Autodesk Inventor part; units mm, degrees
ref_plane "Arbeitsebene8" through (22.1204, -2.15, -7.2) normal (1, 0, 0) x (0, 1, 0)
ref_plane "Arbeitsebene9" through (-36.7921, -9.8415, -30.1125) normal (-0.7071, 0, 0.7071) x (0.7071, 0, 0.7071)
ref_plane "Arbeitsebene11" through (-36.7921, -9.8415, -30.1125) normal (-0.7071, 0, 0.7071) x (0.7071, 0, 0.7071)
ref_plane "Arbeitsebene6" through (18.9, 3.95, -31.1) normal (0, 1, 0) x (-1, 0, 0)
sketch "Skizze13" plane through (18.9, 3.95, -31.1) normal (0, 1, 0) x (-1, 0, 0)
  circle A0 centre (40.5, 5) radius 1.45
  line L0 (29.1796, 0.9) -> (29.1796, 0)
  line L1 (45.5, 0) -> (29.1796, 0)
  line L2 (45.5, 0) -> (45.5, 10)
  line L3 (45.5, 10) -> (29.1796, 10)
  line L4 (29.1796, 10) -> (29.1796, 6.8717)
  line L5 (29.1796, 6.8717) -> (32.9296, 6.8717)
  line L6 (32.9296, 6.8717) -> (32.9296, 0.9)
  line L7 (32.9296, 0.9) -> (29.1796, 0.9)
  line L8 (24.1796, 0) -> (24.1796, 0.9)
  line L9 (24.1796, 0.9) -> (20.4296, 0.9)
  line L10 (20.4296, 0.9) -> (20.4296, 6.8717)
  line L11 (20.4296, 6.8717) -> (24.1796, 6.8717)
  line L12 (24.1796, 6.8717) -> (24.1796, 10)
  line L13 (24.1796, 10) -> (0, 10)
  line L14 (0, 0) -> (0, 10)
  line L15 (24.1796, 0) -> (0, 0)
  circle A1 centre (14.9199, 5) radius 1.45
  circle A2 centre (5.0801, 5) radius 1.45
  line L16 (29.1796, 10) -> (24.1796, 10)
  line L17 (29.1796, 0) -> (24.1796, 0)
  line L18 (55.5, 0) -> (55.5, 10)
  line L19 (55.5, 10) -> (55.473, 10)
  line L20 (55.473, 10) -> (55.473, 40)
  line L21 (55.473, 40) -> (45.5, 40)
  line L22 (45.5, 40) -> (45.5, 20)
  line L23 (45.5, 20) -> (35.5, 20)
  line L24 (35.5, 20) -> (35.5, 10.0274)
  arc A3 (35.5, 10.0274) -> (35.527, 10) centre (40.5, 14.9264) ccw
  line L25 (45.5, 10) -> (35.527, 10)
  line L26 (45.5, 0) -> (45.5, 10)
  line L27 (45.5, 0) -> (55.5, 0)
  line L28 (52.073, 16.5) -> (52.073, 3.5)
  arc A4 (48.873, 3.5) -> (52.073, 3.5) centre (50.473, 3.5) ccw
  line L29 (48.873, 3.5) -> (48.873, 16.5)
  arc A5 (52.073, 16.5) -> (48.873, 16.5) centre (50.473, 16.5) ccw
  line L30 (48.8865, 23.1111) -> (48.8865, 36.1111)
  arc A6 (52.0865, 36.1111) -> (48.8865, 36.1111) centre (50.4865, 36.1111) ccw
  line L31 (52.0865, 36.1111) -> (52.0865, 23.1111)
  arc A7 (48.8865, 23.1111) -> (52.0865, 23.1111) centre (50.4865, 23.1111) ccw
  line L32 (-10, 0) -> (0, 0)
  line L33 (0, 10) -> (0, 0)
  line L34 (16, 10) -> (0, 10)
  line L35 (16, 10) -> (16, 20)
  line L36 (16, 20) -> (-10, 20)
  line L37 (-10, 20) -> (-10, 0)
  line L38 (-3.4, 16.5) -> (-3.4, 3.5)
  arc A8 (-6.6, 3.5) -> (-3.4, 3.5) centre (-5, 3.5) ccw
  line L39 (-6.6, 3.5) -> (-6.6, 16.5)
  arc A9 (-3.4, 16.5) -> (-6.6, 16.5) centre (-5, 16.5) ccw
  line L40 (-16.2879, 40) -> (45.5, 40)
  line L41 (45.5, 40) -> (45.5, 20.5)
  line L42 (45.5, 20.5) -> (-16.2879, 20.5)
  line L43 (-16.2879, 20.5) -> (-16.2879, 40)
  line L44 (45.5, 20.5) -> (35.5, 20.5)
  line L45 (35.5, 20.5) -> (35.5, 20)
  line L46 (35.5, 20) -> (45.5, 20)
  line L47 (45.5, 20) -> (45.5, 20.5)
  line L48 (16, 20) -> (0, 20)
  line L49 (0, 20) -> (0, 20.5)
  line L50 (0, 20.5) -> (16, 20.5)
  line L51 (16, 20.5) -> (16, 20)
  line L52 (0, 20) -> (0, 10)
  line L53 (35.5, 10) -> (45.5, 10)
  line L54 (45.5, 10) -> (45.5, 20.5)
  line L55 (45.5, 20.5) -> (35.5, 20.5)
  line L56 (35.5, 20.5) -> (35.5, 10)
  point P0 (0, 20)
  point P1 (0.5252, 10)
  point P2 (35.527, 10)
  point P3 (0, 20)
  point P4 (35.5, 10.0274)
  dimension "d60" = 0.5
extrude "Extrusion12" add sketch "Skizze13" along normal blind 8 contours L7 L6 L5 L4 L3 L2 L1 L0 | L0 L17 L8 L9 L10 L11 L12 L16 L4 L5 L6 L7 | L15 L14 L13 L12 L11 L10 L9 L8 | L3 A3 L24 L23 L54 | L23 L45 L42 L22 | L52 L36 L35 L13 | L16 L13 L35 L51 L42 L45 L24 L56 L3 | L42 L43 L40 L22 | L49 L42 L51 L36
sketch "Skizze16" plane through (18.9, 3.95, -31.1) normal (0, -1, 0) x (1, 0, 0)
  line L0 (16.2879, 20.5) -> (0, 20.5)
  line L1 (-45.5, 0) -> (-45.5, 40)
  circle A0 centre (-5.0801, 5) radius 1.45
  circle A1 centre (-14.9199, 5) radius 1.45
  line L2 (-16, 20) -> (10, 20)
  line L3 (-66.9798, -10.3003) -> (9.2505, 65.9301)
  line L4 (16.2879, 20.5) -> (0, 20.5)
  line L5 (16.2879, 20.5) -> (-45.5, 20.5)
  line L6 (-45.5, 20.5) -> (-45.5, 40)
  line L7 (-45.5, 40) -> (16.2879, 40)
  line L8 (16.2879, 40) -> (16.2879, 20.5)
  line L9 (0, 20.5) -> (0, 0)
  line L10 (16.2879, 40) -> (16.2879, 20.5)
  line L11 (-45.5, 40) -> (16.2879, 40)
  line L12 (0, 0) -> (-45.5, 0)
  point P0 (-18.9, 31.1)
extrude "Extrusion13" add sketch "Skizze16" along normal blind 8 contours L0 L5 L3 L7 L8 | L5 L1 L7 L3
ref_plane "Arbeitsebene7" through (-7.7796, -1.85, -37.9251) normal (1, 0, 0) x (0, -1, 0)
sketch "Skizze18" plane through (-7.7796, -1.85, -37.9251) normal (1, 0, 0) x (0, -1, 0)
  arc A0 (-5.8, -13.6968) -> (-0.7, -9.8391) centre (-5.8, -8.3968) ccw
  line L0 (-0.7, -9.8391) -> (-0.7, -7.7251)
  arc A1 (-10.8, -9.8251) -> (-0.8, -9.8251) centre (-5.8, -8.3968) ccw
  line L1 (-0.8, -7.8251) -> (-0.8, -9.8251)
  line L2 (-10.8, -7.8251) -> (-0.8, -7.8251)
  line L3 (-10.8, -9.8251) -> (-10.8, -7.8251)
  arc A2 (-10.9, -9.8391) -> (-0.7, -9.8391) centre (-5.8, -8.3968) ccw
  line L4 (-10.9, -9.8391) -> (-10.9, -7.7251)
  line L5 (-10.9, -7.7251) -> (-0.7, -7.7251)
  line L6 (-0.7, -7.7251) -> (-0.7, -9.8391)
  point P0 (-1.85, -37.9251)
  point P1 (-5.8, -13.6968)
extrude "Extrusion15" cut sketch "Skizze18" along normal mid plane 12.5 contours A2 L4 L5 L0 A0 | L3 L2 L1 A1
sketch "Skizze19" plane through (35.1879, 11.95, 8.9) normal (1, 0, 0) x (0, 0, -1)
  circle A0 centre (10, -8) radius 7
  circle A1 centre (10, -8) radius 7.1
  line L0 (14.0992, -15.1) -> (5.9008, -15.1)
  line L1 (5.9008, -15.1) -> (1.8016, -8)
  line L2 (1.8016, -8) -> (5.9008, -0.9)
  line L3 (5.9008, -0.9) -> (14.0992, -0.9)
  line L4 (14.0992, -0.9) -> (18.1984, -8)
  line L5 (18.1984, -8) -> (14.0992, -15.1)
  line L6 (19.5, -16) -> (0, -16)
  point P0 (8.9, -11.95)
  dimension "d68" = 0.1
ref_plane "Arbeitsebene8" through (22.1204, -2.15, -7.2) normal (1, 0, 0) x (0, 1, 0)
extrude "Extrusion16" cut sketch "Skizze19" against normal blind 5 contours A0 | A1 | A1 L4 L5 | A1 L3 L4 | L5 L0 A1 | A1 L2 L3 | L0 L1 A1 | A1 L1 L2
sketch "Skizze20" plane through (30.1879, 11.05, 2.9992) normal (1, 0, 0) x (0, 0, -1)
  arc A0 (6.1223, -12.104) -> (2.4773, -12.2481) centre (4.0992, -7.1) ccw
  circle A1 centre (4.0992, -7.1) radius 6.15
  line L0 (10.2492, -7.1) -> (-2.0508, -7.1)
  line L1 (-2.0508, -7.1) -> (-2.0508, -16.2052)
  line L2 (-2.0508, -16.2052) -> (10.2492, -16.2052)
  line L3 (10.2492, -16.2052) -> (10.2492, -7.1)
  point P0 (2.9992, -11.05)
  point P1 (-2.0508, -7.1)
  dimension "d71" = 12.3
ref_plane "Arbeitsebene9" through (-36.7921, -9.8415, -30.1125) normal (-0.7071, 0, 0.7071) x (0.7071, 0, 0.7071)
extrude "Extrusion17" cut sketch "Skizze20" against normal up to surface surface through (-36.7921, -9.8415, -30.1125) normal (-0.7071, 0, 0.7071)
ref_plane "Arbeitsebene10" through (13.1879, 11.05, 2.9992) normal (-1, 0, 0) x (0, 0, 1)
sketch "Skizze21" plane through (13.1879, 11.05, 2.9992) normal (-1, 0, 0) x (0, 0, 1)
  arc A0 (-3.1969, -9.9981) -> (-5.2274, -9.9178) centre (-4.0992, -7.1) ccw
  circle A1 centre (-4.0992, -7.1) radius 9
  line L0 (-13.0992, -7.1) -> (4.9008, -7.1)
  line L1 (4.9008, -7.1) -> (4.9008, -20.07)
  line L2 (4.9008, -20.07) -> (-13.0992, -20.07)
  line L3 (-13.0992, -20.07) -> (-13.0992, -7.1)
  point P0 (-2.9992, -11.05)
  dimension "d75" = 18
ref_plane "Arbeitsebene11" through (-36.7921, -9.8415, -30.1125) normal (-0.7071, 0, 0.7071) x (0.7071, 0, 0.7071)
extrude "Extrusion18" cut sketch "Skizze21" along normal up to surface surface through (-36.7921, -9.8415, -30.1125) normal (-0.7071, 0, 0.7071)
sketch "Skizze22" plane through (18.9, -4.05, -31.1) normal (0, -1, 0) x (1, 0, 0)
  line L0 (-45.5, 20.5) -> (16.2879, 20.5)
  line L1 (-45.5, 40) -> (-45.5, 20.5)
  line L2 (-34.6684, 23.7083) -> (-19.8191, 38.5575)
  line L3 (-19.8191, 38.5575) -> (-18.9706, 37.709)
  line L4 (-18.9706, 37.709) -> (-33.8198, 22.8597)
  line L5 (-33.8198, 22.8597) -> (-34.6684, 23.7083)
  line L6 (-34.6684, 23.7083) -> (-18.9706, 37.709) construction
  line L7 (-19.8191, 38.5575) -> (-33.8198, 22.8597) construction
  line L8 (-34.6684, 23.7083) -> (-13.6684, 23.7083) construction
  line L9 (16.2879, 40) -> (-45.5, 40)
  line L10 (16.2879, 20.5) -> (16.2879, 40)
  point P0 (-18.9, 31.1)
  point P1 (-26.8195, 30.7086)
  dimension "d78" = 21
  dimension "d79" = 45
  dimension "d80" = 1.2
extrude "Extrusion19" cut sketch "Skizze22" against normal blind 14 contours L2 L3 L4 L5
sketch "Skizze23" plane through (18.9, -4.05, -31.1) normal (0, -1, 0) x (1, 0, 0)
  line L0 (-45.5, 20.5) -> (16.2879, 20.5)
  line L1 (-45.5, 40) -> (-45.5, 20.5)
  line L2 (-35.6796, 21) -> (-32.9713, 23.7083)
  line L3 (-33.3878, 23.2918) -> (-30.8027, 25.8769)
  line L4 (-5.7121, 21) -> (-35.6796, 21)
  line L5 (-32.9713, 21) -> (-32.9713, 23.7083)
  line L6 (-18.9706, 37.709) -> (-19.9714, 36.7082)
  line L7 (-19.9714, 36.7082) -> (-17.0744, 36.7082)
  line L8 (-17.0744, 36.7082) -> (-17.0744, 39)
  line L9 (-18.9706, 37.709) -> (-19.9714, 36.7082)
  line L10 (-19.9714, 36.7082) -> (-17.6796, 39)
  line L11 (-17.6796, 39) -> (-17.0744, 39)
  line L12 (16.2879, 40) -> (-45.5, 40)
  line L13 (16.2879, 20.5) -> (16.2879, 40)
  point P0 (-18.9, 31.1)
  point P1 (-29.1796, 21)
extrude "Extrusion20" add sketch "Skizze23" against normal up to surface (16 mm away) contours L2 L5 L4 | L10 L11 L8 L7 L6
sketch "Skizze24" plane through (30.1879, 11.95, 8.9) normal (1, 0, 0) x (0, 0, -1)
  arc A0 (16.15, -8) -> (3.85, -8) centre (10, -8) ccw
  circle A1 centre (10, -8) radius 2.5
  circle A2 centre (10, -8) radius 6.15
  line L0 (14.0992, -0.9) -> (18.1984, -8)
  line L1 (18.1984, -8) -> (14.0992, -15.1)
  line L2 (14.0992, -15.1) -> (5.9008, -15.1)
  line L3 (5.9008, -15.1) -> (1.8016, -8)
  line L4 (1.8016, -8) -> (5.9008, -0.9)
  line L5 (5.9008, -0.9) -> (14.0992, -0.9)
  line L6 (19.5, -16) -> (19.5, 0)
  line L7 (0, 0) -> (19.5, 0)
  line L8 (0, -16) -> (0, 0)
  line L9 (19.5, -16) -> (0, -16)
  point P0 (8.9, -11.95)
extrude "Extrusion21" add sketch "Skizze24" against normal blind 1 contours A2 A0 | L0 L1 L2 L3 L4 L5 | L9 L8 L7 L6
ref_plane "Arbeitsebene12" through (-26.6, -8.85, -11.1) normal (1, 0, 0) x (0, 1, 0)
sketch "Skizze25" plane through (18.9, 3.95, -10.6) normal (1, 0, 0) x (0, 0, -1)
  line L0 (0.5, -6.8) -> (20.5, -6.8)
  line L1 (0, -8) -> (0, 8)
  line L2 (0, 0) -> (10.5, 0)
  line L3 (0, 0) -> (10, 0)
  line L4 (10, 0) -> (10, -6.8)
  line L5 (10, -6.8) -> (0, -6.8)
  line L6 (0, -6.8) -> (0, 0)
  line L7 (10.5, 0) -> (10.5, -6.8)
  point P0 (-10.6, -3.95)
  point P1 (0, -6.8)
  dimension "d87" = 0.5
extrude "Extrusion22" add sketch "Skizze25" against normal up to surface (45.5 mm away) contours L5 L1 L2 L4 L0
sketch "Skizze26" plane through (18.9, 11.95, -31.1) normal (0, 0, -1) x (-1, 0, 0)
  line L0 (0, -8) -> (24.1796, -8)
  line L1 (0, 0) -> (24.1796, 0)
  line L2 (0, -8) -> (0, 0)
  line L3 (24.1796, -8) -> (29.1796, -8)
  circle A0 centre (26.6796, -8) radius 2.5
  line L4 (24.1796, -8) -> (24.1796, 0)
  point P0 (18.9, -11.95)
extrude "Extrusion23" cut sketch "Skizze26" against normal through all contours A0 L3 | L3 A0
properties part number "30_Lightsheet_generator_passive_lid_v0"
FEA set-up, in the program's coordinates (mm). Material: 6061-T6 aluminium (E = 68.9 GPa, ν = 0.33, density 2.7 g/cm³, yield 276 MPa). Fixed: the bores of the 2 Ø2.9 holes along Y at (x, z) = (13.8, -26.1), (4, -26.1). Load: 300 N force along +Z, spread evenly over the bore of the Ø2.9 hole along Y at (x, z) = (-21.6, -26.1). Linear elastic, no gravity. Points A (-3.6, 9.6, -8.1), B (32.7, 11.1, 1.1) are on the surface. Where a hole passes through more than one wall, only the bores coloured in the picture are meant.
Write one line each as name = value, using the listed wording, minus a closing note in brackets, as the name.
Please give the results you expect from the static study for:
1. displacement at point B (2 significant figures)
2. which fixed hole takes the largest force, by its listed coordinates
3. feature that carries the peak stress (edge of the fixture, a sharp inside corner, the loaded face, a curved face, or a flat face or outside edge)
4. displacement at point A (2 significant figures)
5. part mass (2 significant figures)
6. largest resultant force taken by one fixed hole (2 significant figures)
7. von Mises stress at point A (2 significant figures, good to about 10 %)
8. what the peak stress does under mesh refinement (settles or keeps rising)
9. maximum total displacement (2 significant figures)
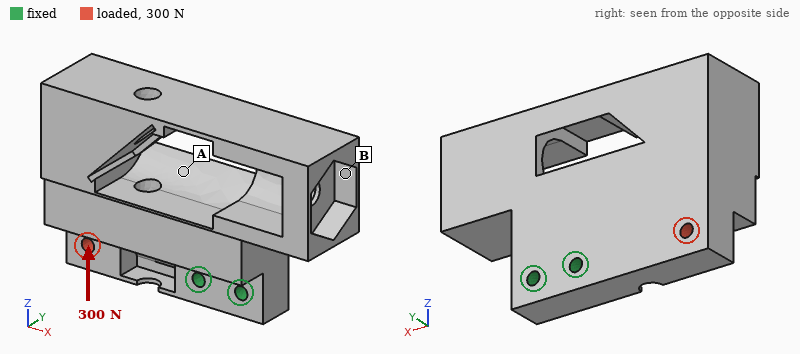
displacement at point B = 13 µm
which fixed hole takes the largest force, by its listed coordinates = (4, -26.1)
feature that carries the peak stress = edge of the fixture
displacement at point A = 6.9 µm
part mass = 53 g
largest resultant force taken by one fixed hole = 900 N
von Mises stress at point A = 8.1 MPa
what the peak stress does under mesh refinement = keeps rising
maximum total displacement = 20 µm
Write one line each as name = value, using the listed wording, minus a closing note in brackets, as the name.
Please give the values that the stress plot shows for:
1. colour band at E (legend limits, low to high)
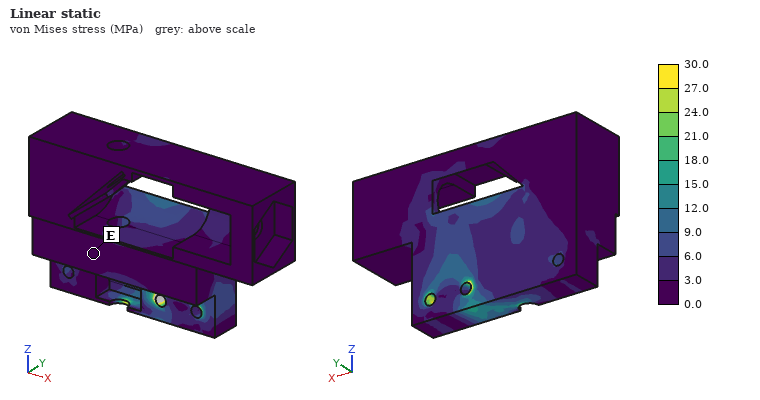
colour band at E = 0.0 to 3.0 MPa
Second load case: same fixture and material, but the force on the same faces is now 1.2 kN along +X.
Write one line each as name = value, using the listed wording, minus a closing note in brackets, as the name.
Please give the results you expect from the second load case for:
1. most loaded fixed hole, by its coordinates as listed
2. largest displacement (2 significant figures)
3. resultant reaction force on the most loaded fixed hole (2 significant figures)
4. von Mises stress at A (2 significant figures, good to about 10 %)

most loaded fixed hole, by its coordinates as listed = (4, -26.1)
largest displacement = 13 µm
resultant reaction force on the most loaded fixed hole = 970 N
von Mises stress at A = 5.9 MPa
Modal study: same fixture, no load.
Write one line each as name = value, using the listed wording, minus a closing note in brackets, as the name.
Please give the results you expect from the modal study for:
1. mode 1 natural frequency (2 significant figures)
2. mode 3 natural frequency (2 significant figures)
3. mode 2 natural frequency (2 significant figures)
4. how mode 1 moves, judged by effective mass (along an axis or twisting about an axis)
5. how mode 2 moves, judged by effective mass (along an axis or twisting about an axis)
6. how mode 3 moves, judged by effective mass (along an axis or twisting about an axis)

mode 1 natural frequency = 2500 Hz
mode 3 natural frequency = 3900 Hz
mode 2 natural frequency = 3800 Hz
how mode 1 moves, judged by effective mass = along Y
how mode 2 moves, judged by effective mass = along X
how mode 3 moves, judged by effective mass = twisting about Z
